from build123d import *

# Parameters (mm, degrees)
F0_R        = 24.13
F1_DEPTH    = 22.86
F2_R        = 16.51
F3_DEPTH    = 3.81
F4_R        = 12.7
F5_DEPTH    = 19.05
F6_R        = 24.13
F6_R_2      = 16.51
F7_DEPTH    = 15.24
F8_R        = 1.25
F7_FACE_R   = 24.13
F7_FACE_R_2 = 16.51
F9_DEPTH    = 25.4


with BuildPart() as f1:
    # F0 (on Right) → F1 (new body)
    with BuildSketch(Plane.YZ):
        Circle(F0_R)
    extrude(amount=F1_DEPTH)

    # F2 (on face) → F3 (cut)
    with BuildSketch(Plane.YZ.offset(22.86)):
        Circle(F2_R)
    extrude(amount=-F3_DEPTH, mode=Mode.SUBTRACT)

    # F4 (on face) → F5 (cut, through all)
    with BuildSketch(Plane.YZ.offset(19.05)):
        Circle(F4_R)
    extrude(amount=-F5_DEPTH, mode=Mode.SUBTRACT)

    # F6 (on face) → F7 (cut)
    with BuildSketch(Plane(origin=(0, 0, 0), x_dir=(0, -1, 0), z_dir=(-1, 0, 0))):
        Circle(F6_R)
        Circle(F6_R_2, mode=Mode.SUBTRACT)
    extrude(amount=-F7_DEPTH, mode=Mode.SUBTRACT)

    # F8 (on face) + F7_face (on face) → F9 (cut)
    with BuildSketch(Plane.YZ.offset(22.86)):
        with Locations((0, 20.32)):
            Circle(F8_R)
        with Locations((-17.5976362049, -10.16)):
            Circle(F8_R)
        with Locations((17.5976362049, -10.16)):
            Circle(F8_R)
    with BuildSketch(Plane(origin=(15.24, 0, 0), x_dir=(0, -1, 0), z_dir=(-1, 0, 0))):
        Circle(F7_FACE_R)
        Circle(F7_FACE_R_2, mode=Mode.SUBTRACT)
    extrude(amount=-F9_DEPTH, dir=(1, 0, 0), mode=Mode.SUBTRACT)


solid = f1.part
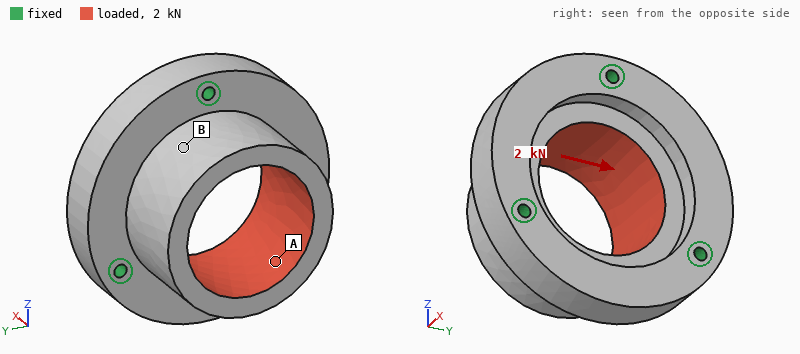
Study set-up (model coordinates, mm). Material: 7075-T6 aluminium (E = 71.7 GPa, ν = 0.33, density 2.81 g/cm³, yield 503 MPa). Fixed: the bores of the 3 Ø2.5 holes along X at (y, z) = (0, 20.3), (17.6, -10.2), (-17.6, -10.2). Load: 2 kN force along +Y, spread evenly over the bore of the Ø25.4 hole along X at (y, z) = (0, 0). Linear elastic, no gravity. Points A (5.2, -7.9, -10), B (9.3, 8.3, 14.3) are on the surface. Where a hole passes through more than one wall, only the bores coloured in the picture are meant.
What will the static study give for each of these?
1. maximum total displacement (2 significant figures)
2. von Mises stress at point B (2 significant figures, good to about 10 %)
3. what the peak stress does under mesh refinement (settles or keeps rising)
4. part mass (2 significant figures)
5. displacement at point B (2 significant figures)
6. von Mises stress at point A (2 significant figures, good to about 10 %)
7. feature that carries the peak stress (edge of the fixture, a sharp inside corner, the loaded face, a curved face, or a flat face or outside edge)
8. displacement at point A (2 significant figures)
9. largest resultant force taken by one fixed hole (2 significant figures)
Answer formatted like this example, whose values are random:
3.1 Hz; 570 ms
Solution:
12 µm; 5.0 MPa; keeps rising; 39 g; 6.7 µm; 11 MPa; edge of the fixture; 4.7 µm; 780 N
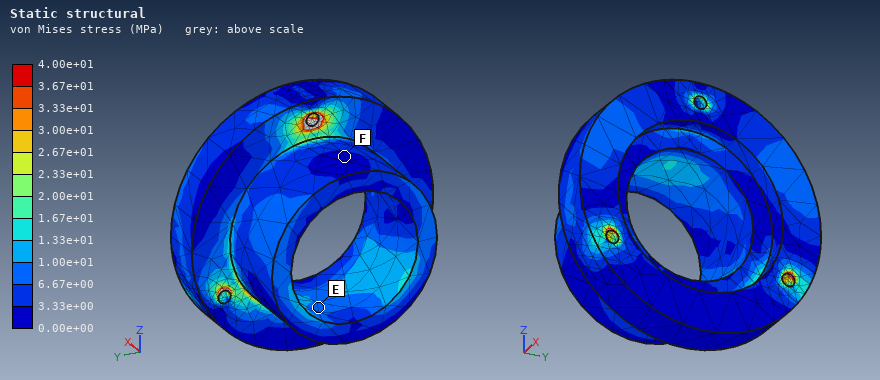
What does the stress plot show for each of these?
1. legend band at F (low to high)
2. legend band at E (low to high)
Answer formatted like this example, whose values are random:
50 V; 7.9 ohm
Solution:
0.00e+00 to 3.33e+00 MPa; 6.67e+00 to 1.00e+01 MPa
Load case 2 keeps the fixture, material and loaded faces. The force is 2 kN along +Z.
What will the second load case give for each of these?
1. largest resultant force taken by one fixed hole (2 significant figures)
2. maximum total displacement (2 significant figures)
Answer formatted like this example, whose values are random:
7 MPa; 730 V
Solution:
780 N; 13 µm
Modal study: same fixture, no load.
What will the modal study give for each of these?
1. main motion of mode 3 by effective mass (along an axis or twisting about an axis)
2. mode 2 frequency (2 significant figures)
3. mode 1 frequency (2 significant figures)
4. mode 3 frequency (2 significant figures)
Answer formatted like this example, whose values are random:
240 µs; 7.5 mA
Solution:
along X; 13 kHz; 13 kHz; 19 kHz
